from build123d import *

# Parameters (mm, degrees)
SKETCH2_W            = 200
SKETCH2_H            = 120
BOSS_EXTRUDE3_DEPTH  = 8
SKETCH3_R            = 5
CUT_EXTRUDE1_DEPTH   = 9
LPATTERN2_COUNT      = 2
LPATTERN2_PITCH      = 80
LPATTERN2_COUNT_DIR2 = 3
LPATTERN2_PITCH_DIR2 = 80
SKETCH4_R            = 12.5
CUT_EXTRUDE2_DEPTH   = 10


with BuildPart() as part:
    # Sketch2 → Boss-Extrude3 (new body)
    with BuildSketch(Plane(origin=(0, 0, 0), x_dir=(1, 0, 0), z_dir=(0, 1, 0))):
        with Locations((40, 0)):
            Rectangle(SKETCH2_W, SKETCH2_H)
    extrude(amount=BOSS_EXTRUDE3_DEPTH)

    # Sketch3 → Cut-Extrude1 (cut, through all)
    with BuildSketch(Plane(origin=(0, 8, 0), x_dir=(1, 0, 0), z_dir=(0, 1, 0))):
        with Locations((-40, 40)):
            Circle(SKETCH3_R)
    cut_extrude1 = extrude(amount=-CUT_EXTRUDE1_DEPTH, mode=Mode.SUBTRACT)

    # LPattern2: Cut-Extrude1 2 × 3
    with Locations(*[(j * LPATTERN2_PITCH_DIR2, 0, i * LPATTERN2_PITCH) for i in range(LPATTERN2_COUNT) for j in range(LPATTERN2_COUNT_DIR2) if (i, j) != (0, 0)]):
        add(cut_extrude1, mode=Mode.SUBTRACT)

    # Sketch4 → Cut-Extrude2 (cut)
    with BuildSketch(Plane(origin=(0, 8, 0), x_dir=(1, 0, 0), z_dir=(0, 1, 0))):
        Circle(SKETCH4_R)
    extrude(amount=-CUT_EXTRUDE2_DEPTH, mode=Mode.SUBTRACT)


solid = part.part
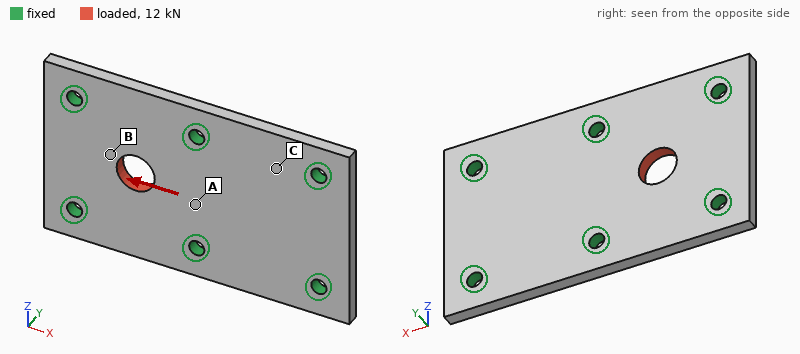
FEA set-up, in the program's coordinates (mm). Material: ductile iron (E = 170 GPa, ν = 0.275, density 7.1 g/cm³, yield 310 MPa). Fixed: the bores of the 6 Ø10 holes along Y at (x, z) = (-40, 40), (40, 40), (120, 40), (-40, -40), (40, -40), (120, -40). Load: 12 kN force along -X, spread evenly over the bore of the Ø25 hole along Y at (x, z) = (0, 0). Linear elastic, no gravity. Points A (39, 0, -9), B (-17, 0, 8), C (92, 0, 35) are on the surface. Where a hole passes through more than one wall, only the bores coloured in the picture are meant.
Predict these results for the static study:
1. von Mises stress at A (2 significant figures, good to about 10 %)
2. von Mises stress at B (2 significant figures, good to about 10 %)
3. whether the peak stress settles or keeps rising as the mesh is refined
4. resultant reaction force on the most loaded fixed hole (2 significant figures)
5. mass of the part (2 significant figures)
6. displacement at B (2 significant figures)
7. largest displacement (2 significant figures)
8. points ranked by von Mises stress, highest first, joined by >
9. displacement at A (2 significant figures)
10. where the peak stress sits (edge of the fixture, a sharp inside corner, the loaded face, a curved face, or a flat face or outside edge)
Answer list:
8.3 MPa
16 MPa
keeps rising
3.0 kN
1.3 kg
4.2 µm
5.0 µm
B > A > C
2.0 µm
edge of the fixture
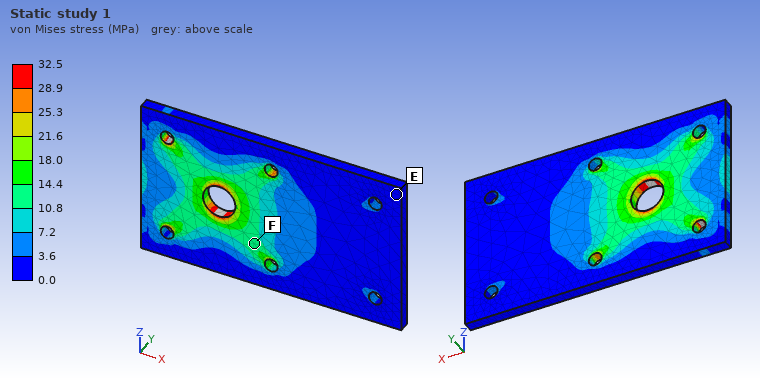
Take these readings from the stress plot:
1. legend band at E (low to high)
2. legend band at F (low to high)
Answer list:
0.0 to 3.6 MPa
10.8 to 14.4 MPa
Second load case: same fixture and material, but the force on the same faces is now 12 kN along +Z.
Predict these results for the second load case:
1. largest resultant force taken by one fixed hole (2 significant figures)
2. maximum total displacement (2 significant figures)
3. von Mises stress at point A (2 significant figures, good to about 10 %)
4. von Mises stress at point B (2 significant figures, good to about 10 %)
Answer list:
3.2 kN
5.1 µm
6.2 MPa
18 MPa
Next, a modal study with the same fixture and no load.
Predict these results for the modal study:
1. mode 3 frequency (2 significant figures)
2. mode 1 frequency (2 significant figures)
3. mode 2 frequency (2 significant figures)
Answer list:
6300 Hz
4700 Hz
4800 Hz
